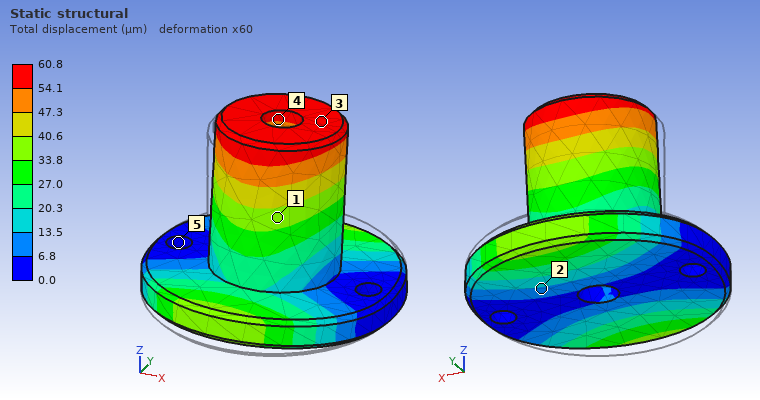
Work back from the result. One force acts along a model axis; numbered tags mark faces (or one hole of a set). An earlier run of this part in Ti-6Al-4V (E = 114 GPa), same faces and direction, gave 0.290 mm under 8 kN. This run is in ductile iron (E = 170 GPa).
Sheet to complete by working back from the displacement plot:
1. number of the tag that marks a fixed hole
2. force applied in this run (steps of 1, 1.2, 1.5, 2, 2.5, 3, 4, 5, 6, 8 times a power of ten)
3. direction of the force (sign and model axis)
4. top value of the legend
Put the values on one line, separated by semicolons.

5; 2.5 kN; +Y; 60.8 µm
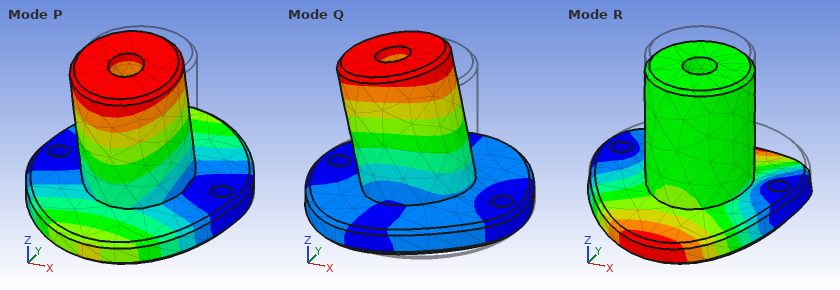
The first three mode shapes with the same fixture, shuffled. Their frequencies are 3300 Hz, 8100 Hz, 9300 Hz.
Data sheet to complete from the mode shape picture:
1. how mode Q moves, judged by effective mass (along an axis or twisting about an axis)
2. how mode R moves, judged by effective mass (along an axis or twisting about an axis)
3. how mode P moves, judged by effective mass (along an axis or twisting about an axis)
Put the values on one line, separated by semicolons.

along X; along Z; along Y
